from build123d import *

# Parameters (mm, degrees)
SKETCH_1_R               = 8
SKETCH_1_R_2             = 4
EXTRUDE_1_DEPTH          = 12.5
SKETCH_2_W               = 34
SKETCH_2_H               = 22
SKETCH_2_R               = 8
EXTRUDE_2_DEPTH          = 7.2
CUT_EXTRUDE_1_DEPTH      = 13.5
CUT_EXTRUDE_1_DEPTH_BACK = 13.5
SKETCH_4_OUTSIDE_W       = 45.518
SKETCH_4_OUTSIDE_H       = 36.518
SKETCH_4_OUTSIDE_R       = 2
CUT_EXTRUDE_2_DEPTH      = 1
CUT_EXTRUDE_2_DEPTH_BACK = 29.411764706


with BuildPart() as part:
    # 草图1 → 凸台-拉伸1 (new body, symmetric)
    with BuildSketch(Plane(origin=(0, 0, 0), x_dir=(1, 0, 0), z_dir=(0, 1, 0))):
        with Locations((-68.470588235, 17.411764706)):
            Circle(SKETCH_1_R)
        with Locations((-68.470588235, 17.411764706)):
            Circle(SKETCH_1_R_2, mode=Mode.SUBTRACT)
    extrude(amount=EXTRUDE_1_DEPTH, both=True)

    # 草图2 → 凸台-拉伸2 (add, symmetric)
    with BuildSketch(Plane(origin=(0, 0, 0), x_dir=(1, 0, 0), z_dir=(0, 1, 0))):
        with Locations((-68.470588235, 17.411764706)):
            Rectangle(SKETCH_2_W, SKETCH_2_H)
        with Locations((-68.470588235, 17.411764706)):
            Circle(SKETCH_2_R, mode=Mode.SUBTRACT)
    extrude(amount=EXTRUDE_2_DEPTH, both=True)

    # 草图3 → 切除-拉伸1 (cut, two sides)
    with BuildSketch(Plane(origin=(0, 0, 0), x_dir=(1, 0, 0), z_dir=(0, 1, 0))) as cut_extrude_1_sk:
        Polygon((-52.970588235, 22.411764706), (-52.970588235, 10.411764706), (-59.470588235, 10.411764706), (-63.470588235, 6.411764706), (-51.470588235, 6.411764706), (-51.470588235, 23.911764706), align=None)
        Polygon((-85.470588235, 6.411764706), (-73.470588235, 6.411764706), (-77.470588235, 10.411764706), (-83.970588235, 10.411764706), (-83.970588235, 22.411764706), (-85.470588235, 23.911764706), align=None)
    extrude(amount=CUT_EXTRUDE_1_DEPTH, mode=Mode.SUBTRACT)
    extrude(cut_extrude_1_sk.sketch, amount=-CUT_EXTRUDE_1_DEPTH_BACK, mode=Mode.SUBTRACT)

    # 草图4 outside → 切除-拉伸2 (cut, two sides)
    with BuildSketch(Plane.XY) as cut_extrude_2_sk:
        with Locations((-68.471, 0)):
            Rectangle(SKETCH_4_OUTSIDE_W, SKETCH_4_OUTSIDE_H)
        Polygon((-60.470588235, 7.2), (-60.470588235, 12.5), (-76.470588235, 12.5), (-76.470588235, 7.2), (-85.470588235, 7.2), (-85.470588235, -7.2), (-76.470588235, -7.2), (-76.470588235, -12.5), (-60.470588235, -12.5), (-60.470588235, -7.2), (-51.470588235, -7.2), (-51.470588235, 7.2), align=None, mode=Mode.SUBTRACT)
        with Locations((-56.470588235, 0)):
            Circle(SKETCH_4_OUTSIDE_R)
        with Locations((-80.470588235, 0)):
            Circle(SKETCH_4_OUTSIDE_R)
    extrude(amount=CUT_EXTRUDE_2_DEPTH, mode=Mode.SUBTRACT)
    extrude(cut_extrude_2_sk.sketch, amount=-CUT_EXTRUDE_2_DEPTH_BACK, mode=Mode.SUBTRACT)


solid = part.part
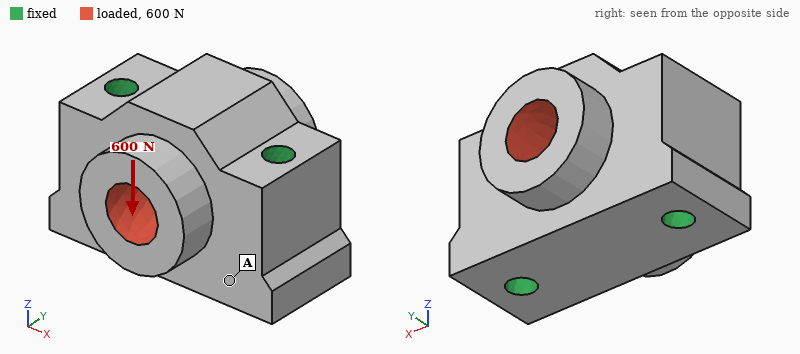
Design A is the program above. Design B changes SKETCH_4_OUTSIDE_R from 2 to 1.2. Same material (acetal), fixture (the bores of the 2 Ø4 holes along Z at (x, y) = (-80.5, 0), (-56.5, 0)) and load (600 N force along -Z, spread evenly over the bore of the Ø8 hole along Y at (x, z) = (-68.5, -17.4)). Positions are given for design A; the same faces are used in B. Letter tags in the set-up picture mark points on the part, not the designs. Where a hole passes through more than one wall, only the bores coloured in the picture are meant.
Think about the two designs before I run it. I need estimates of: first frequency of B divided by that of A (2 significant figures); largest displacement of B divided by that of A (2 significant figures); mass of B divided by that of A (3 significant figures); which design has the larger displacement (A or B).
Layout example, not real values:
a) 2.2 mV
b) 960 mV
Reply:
a) 0.89
b) 1.1
c) 1.03
d) B
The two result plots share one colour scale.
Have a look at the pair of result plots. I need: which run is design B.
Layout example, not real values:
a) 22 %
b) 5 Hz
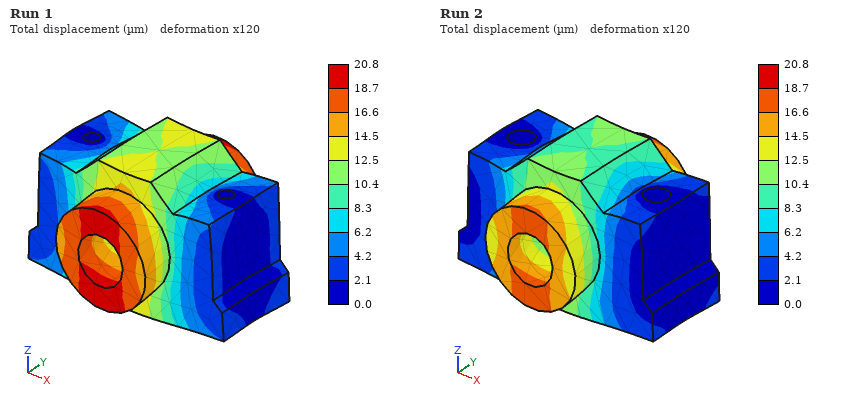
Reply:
a) Run 1
